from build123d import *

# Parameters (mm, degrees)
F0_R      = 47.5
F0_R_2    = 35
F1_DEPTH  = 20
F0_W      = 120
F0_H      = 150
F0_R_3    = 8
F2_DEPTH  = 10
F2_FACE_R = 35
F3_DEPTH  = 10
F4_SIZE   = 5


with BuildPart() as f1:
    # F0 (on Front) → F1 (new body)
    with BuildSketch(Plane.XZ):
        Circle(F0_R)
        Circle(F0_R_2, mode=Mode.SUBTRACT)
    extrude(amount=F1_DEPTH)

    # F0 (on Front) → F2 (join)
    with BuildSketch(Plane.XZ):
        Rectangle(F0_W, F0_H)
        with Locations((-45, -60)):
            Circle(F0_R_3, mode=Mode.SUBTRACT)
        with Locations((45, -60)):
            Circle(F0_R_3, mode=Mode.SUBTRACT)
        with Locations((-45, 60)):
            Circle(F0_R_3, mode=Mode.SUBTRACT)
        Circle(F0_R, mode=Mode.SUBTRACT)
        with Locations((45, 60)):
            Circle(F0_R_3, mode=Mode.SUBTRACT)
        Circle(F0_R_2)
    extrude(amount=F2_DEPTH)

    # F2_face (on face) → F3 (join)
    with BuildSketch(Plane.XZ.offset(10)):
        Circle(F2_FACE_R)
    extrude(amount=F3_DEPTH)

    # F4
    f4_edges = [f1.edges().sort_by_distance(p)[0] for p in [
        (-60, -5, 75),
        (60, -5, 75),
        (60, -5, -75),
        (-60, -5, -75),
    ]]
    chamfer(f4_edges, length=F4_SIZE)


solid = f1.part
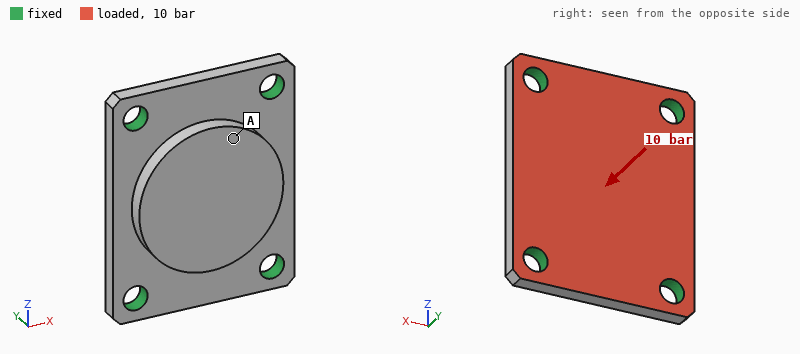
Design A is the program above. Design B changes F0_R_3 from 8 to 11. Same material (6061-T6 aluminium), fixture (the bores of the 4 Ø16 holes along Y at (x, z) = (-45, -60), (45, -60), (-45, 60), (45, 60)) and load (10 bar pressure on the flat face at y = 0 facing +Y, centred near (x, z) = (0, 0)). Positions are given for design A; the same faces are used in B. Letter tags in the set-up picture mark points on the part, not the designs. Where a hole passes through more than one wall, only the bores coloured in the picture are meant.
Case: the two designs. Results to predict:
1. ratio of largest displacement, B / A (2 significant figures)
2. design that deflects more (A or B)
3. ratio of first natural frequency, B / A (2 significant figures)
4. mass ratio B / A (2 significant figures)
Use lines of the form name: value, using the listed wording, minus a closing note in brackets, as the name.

ratio of largest displacement, B / A: 0.76
design that deflects more: A
ratio of first natural frequency, B / A: 1.2
mass ratio B / A: 0.97
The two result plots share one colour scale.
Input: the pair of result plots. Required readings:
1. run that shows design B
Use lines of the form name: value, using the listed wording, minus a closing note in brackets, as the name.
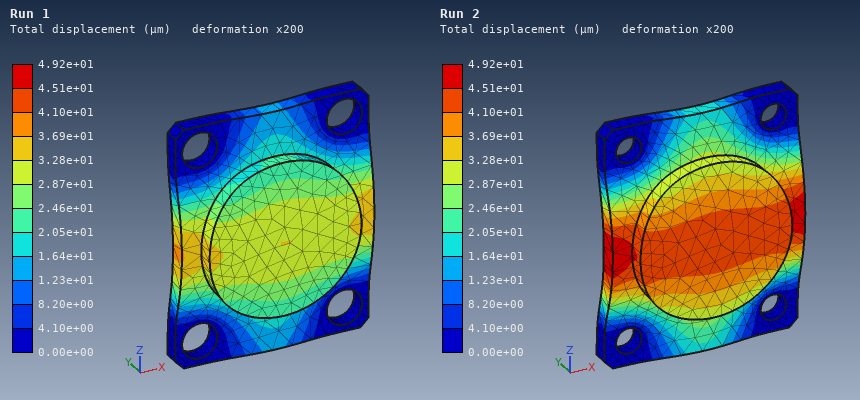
run that shows design B: Run 1
